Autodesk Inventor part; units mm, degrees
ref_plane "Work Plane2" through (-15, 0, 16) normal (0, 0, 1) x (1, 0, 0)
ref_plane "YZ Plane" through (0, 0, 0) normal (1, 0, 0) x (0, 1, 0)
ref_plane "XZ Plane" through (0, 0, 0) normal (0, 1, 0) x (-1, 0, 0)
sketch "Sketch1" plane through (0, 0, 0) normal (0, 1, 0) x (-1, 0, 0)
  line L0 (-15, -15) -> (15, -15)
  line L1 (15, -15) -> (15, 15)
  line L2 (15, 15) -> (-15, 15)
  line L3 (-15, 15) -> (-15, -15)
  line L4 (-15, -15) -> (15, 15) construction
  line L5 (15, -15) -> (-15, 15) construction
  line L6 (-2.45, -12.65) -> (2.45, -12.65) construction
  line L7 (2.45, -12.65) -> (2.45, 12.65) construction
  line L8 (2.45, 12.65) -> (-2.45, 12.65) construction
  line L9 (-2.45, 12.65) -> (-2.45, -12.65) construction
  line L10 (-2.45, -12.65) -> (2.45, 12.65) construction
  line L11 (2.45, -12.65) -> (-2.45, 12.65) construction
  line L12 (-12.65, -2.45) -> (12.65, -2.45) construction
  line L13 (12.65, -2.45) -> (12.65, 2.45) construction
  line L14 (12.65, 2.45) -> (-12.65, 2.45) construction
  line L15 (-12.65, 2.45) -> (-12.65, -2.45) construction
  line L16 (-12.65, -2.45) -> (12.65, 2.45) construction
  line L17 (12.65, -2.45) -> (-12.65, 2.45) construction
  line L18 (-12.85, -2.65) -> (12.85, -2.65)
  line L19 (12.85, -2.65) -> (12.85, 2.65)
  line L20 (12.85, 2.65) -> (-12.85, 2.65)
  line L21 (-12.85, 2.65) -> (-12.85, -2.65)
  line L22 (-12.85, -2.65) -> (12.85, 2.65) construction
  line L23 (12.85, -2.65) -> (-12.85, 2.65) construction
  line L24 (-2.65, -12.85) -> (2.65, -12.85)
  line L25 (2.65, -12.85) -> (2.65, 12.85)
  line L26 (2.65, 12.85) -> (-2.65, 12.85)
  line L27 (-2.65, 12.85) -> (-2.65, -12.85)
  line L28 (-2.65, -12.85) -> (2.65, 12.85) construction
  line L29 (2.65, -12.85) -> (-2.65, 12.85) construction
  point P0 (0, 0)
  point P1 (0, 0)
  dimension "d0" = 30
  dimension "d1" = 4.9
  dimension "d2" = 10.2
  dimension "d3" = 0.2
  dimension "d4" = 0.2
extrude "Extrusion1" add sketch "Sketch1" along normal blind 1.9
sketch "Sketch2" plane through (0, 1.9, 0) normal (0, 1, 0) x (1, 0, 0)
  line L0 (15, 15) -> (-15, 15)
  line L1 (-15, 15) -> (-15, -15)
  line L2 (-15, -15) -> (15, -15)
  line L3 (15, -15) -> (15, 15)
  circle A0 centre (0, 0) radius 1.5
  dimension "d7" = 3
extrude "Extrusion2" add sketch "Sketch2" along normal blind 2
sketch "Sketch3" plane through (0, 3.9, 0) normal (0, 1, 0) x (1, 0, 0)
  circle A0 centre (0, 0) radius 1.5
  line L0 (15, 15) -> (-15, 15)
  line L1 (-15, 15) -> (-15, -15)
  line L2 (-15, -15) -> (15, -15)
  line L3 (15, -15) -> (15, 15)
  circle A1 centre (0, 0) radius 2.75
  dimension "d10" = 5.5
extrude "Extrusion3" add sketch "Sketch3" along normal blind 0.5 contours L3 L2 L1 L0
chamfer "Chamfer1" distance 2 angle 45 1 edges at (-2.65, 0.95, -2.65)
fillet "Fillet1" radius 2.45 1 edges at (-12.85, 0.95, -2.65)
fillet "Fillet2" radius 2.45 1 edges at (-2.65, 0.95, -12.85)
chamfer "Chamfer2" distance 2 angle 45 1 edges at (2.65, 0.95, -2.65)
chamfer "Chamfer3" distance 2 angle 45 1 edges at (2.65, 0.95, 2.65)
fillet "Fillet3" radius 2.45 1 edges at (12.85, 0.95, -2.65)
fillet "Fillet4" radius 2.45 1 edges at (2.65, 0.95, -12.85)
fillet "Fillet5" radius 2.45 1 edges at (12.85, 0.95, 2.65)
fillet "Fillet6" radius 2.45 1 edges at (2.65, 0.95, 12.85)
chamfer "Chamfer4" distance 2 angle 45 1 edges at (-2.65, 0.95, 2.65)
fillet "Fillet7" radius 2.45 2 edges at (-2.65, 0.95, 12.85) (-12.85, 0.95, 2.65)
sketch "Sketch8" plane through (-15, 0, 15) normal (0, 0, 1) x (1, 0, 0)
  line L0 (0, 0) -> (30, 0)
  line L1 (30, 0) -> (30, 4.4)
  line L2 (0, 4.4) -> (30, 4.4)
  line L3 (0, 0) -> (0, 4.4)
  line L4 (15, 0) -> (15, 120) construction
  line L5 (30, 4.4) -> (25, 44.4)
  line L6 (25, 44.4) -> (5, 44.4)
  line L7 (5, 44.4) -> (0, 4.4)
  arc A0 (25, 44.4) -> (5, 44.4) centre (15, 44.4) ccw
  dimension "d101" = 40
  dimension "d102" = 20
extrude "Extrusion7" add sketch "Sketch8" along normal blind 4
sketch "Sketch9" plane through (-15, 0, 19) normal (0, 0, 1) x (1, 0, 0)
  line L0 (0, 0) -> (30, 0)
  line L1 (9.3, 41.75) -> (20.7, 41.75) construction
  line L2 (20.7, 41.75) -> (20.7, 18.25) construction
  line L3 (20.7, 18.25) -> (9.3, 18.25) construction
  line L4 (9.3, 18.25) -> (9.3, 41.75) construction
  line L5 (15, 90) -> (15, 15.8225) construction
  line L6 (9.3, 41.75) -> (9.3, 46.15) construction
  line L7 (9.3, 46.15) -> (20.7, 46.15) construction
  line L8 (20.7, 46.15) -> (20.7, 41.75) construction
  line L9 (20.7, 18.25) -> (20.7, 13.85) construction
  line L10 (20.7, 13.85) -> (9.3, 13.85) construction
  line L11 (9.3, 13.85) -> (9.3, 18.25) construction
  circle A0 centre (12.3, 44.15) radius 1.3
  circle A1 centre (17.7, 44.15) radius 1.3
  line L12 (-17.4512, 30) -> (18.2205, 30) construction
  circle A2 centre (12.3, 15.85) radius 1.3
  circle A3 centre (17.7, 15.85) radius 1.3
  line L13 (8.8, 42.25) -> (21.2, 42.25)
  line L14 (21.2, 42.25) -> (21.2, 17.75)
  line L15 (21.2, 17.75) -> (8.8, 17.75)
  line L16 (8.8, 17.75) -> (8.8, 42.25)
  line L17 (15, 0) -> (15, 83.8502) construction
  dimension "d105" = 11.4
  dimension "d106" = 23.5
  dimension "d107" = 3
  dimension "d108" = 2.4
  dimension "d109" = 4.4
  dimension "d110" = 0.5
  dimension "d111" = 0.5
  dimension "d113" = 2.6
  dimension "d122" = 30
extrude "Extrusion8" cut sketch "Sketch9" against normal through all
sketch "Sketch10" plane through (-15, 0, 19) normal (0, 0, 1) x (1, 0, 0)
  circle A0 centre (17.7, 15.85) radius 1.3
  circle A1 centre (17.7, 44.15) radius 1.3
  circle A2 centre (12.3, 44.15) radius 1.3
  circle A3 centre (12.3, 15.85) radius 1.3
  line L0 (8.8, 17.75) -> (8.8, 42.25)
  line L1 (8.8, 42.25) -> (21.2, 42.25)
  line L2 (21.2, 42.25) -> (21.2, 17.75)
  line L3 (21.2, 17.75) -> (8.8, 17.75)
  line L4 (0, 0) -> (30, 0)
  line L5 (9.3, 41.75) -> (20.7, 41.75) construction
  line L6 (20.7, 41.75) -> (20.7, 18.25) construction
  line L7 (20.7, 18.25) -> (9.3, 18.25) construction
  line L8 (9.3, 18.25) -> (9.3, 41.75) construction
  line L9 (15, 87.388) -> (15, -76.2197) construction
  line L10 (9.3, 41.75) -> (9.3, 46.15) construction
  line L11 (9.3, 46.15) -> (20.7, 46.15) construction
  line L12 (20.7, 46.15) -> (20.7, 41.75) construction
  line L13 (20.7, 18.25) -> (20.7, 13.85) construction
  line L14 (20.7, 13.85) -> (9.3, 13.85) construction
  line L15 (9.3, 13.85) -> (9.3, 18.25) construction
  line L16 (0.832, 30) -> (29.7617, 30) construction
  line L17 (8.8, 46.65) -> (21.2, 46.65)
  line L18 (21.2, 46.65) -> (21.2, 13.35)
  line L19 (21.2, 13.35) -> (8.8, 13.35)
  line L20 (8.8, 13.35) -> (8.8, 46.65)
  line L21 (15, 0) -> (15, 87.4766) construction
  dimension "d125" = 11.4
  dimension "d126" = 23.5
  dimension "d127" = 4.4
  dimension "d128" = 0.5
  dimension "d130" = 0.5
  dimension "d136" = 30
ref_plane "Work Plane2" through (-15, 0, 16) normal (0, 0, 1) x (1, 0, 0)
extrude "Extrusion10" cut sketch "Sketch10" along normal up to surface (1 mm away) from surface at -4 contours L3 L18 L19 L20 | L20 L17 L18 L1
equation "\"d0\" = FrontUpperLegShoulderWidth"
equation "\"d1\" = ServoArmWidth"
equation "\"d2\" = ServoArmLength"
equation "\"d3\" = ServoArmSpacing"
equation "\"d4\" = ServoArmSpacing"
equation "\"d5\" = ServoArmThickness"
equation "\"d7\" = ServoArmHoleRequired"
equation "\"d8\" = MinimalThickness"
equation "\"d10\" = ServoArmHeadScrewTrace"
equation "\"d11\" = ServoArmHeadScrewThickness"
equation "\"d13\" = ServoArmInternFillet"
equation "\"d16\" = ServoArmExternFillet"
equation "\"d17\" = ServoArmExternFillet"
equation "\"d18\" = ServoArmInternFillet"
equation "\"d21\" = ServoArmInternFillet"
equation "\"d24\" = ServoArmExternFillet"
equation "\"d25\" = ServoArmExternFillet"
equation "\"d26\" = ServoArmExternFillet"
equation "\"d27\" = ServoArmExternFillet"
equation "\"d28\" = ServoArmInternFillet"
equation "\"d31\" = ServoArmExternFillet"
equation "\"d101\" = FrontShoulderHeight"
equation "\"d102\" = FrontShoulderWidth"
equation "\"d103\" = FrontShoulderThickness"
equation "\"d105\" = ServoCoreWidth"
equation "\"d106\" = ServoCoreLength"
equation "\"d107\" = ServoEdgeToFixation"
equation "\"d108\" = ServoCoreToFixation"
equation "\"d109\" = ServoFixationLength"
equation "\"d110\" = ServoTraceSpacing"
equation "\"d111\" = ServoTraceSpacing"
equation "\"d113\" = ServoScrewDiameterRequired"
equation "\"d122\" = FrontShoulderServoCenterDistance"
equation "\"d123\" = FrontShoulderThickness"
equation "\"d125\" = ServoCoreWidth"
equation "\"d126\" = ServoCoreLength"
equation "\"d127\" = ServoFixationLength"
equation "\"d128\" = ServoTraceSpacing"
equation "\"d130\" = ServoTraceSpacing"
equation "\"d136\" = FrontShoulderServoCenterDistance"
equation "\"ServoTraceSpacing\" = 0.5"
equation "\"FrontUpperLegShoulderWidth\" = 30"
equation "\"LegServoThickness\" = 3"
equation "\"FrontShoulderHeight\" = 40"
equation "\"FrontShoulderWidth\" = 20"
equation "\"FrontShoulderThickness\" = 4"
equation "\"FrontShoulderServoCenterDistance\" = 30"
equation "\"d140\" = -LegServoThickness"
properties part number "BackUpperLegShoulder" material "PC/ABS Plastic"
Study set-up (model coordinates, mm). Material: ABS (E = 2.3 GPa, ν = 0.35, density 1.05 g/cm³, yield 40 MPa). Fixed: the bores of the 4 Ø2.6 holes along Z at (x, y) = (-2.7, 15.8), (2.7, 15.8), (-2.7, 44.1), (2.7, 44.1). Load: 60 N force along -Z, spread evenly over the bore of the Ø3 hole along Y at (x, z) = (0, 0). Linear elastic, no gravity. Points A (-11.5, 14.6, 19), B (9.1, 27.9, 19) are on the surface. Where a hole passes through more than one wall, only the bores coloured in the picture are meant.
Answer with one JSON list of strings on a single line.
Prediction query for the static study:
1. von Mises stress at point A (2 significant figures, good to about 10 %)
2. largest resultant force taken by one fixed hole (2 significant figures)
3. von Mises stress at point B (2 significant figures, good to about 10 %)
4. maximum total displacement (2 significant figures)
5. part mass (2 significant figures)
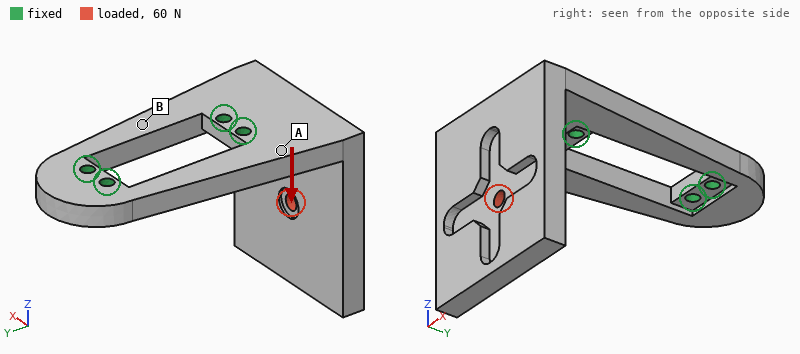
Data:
["5.5 MPa", "35 N", "2.6 MPa", "0.77 mm", "7.6 g"]
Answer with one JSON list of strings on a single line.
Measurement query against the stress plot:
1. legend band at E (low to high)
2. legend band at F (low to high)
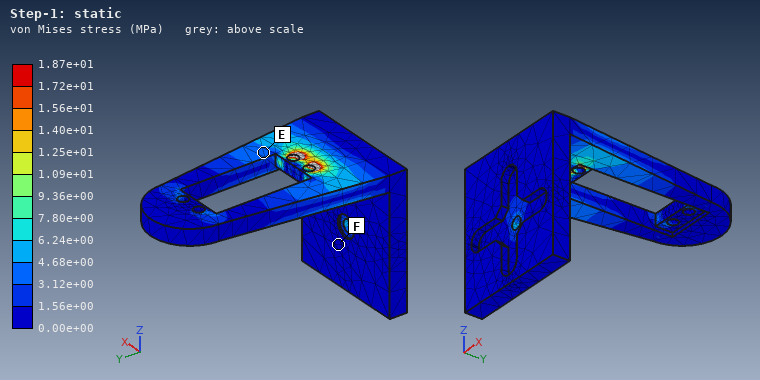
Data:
["3.12e+00 to 4.68e+00 MPa", "0.00e+00 to 1.56e+00 MPa"]
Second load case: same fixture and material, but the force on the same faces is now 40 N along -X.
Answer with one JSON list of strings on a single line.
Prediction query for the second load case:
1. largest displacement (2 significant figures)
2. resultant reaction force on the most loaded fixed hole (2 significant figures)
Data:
["0.68 mm", "77 N"]
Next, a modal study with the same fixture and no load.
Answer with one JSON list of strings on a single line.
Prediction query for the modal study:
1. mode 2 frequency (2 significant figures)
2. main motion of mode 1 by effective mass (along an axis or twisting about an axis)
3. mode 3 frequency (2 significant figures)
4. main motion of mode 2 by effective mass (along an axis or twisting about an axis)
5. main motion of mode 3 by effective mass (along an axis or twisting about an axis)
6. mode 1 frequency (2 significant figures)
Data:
["730 Hz", "along Y", "1700 Hz", "along X", "along Z", "500 Hz"]
